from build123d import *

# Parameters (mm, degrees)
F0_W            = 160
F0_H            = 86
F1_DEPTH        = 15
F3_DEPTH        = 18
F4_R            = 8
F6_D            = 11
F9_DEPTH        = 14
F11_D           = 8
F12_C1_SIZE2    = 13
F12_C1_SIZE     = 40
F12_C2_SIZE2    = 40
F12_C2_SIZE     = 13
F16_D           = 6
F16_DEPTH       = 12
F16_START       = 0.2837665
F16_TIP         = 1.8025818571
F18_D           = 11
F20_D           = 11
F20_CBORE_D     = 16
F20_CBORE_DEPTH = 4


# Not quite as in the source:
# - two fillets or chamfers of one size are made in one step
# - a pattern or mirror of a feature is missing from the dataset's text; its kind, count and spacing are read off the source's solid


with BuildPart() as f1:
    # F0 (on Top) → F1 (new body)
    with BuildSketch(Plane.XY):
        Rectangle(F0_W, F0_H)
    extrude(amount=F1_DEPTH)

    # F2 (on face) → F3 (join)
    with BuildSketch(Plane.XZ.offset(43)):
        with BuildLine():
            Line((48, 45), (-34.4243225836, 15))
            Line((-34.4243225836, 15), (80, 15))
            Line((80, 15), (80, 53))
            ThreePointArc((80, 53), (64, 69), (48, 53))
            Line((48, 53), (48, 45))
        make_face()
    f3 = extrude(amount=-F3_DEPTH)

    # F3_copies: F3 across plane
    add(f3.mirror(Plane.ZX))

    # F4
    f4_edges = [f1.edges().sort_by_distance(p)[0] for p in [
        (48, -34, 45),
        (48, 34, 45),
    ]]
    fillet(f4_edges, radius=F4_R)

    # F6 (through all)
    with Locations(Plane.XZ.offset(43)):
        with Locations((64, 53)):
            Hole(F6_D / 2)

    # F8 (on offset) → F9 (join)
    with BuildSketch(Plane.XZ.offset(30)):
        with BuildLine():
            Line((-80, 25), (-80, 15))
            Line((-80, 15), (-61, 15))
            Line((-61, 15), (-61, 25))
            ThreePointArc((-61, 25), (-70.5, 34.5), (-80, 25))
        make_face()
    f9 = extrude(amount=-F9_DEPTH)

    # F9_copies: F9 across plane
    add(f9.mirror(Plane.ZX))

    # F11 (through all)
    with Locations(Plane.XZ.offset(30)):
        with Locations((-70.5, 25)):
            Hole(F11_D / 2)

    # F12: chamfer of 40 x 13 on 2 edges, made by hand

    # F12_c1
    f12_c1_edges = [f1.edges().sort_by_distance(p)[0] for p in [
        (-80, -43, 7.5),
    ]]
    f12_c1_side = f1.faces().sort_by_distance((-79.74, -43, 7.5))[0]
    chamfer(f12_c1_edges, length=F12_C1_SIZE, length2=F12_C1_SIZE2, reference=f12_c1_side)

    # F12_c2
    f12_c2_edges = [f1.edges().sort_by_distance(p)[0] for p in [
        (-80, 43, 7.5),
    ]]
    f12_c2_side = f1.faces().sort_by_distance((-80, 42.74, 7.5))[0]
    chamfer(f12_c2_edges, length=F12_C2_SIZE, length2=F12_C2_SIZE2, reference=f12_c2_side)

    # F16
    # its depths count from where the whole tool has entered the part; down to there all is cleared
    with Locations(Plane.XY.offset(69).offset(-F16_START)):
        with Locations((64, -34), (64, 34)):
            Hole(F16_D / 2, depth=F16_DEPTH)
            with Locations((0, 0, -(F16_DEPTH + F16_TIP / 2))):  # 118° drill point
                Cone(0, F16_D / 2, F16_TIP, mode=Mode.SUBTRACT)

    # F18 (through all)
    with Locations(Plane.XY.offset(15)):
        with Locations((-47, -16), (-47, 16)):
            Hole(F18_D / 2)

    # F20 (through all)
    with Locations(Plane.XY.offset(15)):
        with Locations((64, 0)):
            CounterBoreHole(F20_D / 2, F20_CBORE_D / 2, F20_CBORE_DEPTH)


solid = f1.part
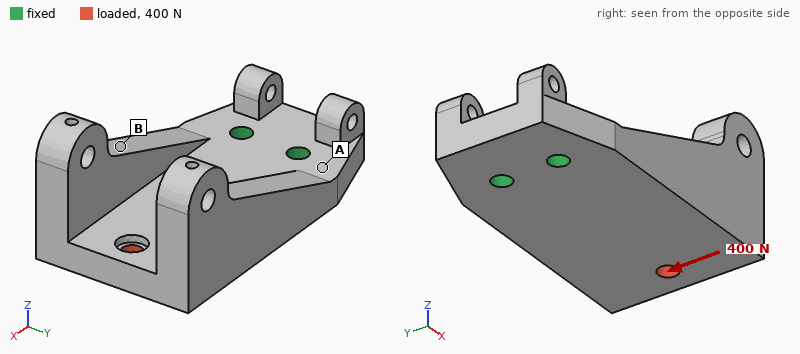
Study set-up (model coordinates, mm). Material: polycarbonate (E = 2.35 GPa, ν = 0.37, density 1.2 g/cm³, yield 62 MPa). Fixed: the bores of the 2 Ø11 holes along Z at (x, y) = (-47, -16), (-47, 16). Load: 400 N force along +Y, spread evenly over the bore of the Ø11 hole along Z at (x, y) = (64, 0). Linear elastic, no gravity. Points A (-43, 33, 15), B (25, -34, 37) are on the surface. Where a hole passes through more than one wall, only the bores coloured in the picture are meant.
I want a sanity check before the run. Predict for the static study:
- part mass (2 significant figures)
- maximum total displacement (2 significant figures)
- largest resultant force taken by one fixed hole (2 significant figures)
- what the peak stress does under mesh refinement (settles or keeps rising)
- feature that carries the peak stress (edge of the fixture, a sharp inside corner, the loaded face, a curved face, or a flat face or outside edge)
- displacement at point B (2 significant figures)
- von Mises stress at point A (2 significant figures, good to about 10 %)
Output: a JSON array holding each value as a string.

["360 g", "0.26 mm", "1.1 kN", "keeps rising", "edge of the fixture", "0.12 mm", "1.8 MPa"]
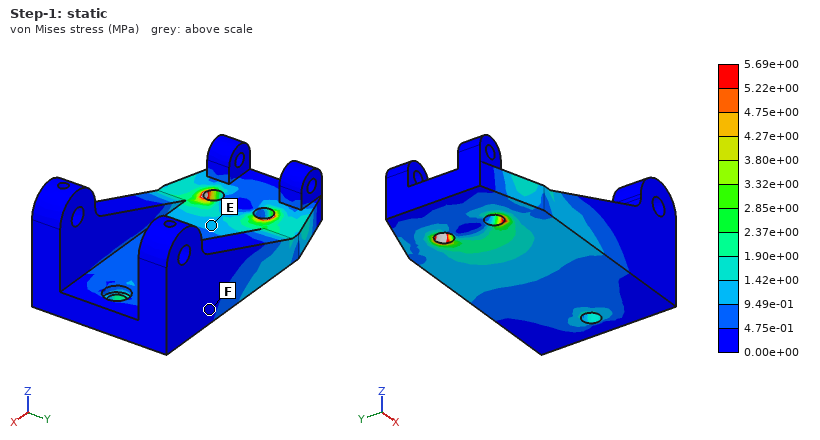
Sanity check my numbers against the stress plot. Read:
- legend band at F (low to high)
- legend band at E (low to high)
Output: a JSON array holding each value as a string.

["0.00e+00 to 4.75e-01 MPa", "9.49e-01 to 1.42e+00 MPa"]
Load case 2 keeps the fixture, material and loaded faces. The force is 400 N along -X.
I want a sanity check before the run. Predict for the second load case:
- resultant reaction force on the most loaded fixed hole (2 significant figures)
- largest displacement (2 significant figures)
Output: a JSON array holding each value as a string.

["200 N", "92 µm"]
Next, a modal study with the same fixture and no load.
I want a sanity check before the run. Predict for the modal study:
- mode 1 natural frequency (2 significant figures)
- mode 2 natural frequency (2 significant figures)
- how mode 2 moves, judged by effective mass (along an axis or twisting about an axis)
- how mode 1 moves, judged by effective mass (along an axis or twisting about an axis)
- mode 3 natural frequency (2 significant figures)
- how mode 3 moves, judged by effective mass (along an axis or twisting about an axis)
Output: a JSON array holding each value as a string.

["170 Hz", "340 Hz", "along Y", "along Z", "550 Hz", "along Y"]
